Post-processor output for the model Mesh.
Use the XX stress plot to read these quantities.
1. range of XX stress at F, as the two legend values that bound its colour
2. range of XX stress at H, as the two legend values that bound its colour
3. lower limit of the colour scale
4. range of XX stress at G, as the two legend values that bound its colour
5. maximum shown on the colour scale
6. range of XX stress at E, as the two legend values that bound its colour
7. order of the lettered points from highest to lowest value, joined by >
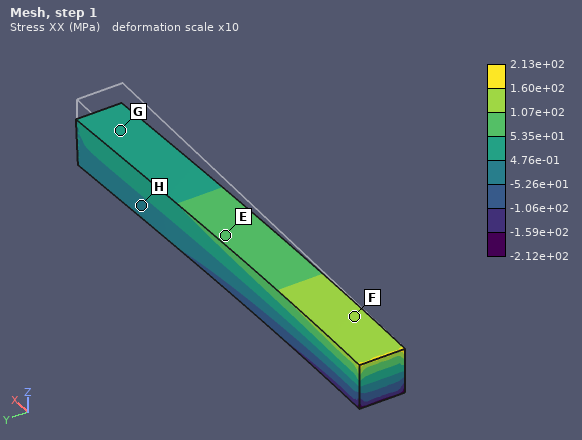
1.07e+02 to 1.60e+02 MPa
-5.26e+01 to 4.76e-01 MPa
-2.12e+02 MPa
4.76e-01 to 5.35e+01 MPa
2.13e+02 MPa
5.35e+01 to 1.07e+02 MPa
F > E > G > H
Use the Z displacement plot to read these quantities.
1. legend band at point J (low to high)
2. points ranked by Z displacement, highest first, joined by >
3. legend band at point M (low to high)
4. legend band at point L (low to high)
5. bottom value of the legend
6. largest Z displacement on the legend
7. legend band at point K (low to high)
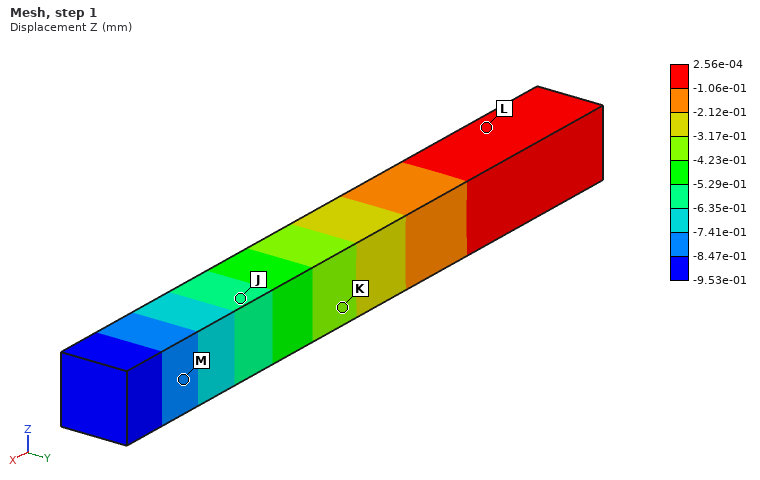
-6.35e-01 to -5.29e-01 mm
L > K > J > M
-8.47e-01 to -7.41e-01 mm
-1.06e-01 to 2.56e-04 mm
-9.53e-01 mm
2.56e-04 mm
-4.23e-01 to -3.17e-01 mm
